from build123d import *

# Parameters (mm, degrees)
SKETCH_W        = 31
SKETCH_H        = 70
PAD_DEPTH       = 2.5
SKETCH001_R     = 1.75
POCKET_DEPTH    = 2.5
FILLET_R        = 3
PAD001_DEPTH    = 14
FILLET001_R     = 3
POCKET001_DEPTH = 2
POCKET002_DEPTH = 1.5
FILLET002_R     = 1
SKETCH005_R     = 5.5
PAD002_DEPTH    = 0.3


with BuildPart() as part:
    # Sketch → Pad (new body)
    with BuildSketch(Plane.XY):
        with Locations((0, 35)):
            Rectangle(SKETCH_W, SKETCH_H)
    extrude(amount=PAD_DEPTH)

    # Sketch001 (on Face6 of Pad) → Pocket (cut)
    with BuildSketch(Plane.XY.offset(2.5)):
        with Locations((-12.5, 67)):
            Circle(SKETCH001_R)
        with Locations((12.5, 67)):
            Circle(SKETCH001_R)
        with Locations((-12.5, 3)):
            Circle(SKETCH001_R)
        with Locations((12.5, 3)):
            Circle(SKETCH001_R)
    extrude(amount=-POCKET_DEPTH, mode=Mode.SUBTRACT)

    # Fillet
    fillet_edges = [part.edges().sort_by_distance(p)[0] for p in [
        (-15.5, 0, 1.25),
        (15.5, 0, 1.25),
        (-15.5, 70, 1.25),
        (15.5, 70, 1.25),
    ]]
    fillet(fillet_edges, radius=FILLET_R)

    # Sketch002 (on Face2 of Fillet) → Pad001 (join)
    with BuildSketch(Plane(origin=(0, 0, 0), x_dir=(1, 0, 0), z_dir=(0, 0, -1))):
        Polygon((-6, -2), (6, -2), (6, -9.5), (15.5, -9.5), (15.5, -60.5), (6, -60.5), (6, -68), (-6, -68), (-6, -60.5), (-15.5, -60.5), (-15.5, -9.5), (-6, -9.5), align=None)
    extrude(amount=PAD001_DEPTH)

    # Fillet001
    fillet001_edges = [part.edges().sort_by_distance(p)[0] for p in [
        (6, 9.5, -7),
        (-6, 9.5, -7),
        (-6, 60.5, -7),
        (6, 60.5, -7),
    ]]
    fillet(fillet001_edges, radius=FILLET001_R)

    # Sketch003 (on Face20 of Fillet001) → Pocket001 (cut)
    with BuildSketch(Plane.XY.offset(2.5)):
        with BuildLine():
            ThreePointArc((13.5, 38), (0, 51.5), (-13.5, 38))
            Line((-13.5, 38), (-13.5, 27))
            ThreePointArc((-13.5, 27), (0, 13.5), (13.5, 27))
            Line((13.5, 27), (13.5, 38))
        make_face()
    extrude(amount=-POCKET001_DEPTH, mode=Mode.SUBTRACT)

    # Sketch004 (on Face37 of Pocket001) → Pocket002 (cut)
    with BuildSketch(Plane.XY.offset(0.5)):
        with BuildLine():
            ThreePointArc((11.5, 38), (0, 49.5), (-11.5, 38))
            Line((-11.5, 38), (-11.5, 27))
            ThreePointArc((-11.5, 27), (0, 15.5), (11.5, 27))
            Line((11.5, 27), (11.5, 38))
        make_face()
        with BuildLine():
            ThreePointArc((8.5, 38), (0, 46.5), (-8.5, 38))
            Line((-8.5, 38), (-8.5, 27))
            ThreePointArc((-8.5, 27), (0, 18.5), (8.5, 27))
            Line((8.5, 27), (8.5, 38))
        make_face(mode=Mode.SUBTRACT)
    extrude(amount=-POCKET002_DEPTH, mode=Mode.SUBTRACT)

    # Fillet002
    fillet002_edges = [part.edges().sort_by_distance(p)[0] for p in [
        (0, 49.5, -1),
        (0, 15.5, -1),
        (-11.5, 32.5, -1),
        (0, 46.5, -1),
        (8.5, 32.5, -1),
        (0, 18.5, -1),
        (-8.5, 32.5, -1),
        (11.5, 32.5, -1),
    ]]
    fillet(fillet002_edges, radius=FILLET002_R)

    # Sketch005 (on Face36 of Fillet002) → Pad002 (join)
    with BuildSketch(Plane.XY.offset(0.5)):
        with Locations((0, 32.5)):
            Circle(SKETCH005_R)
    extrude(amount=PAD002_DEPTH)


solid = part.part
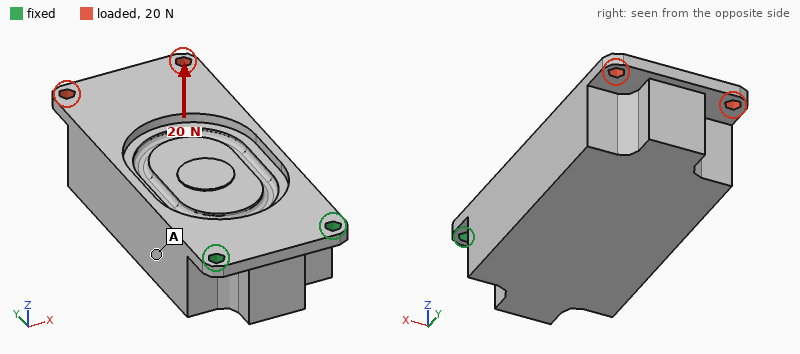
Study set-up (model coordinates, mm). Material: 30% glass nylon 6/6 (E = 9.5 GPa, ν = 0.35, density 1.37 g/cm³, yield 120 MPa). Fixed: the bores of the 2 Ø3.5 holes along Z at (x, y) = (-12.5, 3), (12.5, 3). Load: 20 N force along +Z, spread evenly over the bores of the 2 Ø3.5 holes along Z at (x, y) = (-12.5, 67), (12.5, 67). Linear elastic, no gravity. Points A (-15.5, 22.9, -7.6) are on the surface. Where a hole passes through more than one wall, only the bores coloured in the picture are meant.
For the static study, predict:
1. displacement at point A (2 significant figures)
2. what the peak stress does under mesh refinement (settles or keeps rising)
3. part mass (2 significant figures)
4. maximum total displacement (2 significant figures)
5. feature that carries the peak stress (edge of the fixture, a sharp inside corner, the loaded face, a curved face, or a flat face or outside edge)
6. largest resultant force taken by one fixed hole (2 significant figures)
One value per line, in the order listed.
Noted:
0.26 mm
keeps rising
38 g
0.88 mm
edge of the fixture
26 N
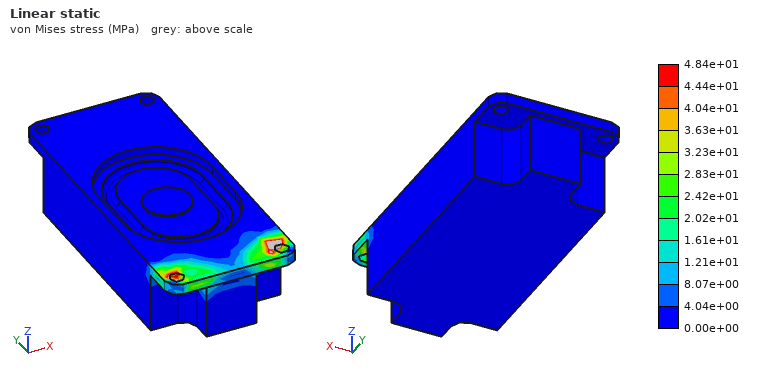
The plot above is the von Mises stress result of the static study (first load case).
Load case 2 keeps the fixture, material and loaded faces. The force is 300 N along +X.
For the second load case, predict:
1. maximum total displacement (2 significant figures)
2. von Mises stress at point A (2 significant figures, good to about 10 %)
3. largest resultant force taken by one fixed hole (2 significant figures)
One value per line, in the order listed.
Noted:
0.35 mm
4.5 MPa
770 N
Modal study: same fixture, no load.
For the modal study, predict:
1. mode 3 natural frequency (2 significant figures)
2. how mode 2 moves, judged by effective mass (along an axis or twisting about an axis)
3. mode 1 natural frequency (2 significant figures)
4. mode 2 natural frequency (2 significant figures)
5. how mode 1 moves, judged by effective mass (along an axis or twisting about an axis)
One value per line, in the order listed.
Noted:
2400 Hz
along X
220 Hz
1500 Hz
along Z
